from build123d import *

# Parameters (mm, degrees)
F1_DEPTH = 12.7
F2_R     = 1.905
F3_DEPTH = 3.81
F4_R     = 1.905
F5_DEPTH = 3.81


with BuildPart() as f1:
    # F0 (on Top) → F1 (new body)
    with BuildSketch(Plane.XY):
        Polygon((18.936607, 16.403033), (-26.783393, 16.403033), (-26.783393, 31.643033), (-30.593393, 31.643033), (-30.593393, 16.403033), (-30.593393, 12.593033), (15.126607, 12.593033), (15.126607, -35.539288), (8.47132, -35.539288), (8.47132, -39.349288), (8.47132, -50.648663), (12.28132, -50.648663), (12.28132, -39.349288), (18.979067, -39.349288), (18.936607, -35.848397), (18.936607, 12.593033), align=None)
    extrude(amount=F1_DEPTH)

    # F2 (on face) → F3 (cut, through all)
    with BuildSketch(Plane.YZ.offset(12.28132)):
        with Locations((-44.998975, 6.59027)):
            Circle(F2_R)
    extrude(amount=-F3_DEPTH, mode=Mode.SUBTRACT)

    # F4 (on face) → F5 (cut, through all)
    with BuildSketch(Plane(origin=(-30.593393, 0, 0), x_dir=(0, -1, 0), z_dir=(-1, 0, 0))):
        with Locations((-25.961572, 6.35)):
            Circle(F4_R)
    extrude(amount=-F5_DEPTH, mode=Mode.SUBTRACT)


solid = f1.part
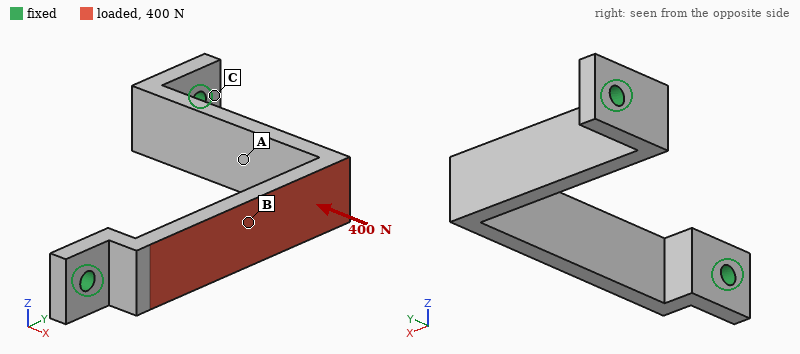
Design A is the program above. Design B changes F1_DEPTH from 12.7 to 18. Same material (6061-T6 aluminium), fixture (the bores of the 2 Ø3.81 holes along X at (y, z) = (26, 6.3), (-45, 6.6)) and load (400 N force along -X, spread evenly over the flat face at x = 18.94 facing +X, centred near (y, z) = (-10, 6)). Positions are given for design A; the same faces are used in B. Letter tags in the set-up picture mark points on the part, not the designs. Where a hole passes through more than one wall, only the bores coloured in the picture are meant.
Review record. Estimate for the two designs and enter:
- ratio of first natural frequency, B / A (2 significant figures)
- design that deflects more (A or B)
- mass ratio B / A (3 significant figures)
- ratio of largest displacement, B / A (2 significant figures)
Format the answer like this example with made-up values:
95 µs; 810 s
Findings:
1.0; A; 1.42; 0.77
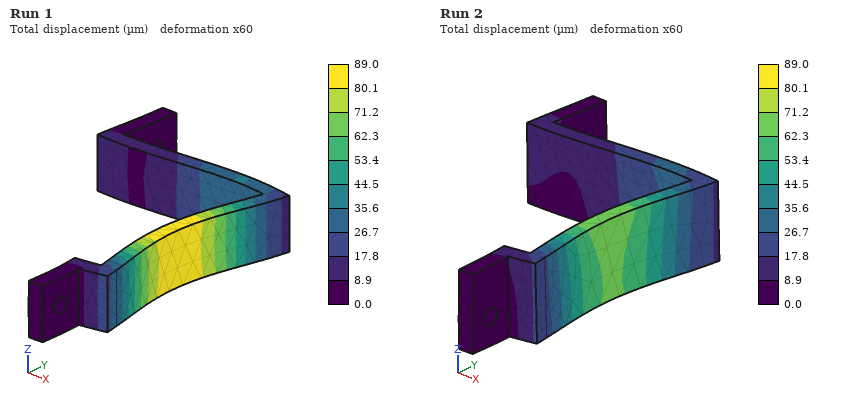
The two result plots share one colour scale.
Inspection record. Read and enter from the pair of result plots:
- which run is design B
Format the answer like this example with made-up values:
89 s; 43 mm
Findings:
Run 2
